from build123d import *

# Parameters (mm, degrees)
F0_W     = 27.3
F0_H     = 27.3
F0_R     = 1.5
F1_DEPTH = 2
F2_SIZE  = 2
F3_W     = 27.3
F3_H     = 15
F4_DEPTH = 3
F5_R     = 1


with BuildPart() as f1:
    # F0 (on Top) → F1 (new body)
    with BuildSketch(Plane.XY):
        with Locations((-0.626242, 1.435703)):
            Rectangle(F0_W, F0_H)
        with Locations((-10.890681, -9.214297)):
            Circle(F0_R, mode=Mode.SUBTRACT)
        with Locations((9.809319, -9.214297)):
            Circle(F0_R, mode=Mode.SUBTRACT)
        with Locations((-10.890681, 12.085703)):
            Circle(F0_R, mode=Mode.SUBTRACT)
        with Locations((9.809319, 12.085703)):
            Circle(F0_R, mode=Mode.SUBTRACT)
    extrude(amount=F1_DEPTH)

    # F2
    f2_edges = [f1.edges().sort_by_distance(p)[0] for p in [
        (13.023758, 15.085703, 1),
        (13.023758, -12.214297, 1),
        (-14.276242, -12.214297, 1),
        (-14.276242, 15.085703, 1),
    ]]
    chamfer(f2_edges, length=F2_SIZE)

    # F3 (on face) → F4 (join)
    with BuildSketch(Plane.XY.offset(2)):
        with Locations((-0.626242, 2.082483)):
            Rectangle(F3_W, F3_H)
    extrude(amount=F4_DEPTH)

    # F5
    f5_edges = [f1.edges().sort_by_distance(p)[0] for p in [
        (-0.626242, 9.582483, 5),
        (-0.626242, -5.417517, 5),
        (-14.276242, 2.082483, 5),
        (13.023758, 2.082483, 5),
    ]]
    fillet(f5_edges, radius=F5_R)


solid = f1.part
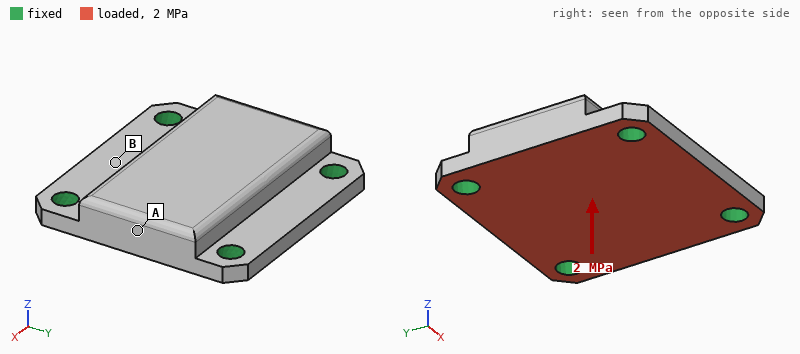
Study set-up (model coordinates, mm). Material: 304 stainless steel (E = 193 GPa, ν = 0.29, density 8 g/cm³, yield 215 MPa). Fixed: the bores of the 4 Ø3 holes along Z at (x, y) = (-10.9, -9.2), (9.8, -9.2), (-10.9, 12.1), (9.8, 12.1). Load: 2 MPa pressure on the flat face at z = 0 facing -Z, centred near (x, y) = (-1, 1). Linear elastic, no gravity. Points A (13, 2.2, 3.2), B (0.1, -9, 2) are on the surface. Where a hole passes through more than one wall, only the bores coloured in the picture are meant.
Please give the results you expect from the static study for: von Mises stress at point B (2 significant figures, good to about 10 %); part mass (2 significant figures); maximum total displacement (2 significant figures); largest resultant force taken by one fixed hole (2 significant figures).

27 MPa
21 g
5.1 µm
390 N
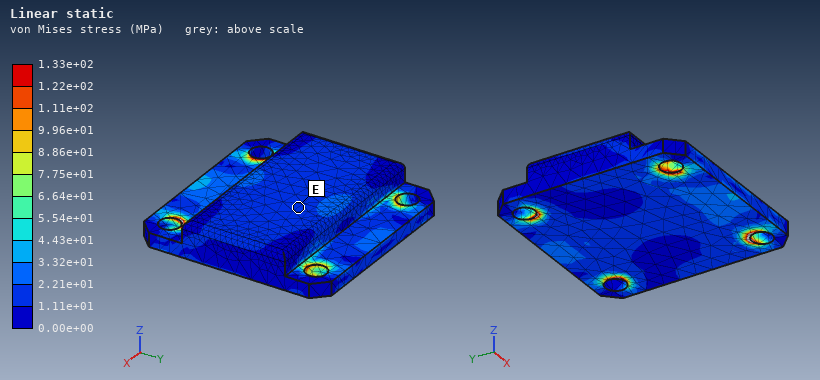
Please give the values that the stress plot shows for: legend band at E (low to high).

1.11e+01 to 2.21e+01 MPa
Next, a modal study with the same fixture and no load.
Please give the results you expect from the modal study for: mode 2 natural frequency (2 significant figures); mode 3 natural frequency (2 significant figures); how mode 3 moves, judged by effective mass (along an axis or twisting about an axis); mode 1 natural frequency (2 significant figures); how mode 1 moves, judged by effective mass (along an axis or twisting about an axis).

32 kHz
35 kHz
twisting about X
22 kHz
along Z
